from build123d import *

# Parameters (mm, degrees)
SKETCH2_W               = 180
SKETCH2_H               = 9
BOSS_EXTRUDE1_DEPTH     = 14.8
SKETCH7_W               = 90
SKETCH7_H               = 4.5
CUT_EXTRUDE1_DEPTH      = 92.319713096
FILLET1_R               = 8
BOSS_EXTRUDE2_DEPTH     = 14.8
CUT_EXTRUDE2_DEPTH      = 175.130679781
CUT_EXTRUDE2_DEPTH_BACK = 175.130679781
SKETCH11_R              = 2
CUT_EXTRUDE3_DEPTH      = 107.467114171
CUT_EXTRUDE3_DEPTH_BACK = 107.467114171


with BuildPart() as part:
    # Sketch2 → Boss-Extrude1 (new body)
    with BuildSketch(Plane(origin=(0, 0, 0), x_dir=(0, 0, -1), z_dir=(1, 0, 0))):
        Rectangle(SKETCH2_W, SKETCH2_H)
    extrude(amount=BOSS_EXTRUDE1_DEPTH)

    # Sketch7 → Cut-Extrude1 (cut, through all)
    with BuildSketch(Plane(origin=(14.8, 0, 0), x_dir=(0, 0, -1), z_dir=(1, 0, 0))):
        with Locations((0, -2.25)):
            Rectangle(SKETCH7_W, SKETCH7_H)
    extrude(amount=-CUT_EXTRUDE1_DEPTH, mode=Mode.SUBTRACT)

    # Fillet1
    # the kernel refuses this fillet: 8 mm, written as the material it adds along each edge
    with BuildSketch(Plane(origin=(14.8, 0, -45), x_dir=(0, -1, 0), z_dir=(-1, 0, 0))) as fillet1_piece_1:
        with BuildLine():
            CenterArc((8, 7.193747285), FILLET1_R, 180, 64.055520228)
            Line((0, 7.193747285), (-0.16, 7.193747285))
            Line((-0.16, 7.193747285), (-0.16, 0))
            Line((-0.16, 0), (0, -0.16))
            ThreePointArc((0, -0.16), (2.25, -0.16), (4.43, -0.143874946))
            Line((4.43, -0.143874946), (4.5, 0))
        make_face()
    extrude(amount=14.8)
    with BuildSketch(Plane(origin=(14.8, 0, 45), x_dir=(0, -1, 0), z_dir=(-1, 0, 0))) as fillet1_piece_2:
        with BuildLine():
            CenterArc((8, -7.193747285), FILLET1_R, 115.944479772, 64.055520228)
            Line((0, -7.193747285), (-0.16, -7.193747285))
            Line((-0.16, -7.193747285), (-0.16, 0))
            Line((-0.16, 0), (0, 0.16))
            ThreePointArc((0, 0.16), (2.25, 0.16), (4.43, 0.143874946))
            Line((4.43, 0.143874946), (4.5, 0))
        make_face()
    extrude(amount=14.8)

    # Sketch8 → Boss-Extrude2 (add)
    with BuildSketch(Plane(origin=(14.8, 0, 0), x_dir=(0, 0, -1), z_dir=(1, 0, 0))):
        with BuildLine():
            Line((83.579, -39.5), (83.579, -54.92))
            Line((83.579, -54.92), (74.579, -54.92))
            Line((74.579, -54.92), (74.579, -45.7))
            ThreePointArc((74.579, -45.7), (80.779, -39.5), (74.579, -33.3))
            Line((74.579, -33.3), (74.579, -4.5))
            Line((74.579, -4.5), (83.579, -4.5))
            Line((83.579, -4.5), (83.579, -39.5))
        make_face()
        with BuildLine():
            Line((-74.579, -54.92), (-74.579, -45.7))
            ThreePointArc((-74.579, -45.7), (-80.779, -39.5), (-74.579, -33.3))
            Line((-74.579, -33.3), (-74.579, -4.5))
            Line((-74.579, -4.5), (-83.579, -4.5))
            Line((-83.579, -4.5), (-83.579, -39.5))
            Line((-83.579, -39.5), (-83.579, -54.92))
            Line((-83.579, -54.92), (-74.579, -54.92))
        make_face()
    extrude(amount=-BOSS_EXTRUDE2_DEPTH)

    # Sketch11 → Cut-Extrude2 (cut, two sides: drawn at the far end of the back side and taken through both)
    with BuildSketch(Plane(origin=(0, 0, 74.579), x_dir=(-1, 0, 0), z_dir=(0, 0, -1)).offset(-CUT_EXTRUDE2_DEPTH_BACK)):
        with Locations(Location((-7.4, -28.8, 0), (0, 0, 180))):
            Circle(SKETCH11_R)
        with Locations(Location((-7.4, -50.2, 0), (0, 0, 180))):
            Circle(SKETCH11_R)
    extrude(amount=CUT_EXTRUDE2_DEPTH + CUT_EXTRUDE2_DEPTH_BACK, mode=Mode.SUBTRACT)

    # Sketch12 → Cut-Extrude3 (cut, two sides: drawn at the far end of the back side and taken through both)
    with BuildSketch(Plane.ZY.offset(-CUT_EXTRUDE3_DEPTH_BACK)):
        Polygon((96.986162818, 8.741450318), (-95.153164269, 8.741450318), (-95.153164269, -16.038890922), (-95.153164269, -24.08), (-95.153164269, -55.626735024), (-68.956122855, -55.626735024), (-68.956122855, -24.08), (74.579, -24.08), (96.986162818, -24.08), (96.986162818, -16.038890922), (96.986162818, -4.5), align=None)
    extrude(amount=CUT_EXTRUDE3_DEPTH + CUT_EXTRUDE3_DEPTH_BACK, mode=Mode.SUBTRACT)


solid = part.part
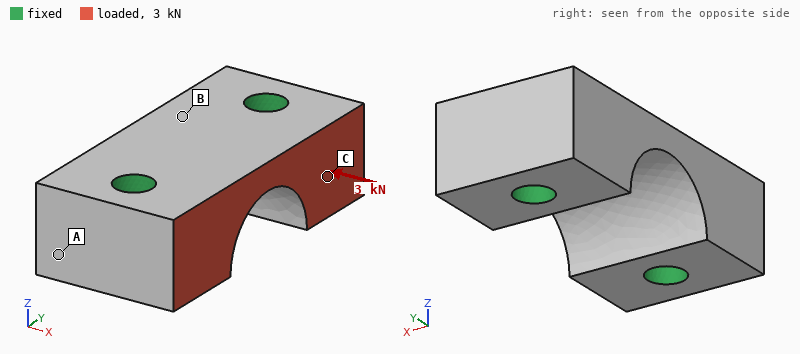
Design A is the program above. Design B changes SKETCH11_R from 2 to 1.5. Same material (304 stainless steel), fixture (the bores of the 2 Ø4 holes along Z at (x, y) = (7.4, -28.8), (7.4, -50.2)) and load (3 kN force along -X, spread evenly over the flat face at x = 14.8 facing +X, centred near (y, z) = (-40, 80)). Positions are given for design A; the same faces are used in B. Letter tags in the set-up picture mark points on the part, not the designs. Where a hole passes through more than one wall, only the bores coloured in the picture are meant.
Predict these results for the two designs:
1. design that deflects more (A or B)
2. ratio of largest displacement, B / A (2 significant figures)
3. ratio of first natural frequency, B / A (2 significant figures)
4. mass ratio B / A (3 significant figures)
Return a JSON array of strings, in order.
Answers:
["B", "1.2", "0.85", "1.03"]
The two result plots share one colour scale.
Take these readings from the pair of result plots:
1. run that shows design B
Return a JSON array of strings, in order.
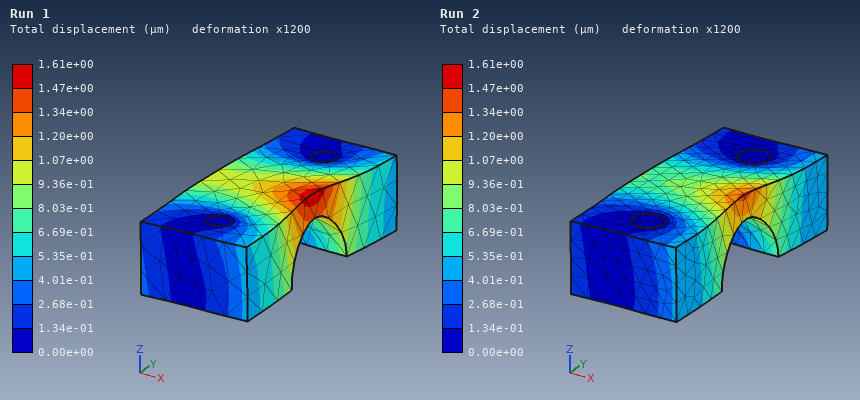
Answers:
["Run 1"]
